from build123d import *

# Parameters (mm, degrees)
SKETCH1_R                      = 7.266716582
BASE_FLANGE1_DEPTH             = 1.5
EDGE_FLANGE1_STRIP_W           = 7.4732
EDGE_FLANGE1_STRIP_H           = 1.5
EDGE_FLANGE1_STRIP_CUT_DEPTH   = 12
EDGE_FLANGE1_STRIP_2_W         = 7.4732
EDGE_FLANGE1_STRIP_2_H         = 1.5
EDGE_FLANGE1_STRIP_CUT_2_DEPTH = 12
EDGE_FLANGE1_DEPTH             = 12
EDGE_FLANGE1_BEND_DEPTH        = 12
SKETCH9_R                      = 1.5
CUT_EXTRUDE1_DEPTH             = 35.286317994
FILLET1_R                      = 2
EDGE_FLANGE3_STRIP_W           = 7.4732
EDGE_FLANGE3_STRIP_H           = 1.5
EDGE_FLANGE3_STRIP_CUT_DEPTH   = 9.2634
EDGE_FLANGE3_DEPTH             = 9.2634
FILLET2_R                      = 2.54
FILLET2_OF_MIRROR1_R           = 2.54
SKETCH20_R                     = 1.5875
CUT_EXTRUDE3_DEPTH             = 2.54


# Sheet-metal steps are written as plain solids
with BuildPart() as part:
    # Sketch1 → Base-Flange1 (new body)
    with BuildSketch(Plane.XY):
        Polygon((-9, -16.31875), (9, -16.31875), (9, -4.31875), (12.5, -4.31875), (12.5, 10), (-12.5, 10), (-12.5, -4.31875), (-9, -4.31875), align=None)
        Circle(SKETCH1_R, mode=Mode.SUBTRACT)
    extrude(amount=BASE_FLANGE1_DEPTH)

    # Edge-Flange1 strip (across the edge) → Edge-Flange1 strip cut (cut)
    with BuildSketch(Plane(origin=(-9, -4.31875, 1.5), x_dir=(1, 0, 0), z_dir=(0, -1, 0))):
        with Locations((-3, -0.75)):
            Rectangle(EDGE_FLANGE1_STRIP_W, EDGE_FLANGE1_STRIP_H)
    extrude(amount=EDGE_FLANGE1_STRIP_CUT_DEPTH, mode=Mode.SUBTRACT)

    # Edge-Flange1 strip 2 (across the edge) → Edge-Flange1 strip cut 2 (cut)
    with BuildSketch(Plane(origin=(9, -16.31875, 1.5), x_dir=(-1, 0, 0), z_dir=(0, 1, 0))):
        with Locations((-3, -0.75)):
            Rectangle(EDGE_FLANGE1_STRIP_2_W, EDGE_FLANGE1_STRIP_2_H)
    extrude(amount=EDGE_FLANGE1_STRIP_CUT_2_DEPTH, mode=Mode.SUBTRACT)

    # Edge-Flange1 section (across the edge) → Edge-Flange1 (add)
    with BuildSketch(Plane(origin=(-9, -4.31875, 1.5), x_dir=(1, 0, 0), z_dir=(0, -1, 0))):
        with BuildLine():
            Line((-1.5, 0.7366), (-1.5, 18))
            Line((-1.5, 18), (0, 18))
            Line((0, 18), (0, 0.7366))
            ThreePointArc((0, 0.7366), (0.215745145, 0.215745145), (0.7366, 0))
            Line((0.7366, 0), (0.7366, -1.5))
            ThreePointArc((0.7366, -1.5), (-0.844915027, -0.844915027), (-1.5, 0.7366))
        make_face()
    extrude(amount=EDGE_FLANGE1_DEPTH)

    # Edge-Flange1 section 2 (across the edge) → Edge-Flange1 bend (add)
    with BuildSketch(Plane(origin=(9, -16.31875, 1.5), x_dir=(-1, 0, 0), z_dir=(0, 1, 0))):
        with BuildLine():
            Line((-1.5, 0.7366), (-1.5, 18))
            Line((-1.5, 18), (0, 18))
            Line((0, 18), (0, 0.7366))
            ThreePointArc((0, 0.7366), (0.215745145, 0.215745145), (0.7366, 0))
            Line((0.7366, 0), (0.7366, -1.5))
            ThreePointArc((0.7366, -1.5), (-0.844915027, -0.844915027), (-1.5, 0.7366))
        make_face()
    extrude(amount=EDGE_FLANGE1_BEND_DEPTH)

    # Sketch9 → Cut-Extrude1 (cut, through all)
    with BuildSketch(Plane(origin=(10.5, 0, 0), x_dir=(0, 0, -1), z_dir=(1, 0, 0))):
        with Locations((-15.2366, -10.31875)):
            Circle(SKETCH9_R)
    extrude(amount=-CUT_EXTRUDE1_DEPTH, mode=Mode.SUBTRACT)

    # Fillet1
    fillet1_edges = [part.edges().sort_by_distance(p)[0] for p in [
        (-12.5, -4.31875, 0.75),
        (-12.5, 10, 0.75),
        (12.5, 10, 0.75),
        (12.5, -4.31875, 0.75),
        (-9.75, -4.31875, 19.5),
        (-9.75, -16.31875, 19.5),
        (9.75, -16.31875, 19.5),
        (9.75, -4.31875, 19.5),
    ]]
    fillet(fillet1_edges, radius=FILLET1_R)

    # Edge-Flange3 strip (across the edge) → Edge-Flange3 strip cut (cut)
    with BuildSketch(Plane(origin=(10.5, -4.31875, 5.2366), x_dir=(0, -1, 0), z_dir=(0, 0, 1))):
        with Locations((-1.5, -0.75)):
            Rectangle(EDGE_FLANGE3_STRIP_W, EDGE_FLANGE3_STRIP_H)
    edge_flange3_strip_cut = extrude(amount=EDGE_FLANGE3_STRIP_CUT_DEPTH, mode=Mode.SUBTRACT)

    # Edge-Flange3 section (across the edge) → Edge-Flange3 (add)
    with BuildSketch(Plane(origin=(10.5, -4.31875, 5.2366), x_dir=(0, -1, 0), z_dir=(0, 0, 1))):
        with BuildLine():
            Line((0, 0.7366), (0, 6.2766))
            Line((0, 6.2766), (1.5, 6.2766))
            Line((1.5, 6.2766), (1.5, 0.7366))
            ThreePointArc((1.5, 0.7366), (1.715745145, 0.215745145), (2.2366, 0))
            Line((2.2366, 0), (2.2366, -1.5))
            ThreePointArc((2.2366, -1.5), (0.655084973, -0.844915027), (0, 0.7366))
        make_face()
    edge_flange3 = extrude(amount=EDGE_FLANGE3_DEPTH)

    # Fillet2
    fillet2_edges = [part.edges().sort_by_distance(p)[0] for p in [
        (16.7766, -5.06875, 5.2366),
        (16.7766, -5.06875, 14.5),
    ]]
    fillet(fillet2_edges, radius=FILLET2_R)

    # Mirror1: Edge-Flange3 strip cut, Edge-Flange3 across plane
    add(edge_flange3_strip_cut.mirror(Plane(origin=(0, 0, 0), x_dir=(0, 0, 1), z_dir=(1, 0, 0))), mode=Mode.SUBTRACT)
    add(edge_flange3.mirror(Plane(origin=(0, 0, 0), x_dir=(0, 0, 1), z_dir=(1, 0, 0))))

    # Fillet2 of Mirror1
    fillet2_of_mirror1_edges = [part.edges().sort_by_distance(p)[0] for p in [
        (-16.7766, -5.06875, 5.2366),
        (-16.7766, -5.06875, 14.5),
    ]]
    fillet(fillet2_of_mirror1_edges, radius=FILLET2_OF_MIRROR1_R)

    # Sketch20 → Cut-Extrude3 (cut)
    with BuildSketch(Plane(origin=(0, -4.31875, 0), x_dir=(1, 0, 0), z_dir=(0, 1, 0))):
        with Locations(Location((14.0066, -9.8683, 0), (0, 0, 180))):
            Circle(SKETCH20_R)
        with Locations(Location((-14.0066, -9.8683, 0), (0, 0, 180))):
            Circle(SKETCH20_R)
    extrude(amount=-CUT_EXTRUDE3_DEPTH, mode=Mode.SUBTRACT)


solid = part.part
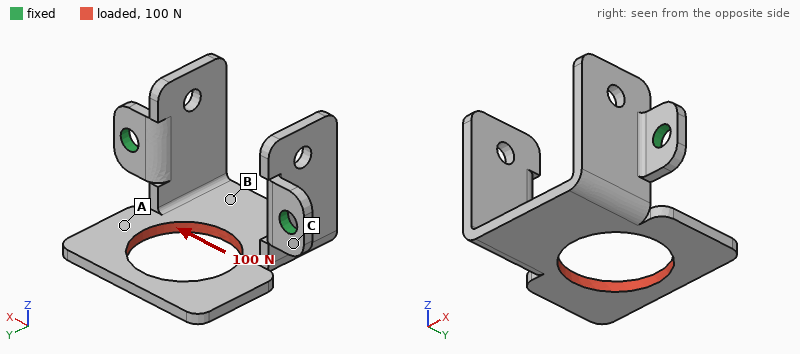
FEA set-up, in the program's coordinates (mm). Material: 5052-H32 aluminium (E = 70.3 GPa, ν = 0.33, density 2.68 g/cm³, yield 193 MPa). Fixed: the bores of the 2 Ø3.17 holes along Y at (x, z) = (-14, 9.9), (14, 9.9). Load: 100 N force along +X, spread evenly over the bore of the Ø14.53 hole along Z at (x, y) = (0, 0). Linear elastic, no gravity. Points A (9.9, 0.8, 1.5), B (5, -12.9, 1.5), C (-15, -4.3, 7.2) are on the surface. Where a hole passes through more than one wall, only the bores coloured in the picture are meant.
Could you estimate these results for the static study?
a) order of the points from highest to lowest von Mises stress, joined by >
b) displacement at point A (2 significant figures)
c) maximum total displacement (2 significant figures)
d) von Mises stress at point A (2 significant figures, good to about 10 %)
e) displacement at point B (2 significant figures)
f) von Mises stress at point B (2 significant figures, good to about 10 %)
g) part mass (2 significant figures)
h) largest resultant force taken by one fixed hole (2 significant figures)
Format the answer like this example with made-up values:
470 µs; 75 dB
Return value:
A > B > C; 44 µm; 66 µm; 25 MPa; 13 µm; 14 MPa; 3.7 g; 57 N
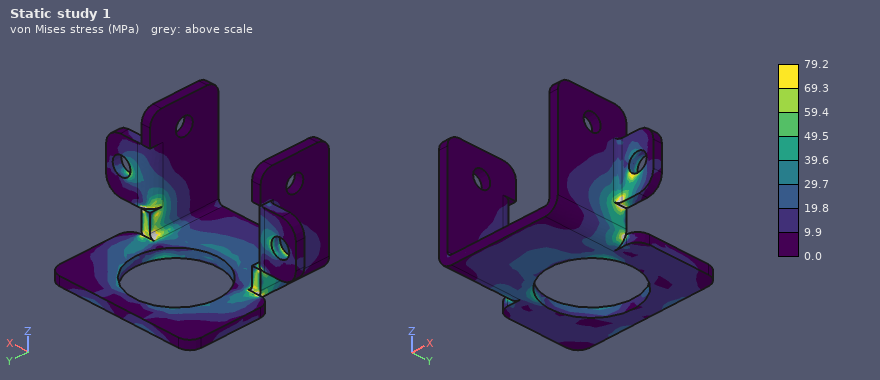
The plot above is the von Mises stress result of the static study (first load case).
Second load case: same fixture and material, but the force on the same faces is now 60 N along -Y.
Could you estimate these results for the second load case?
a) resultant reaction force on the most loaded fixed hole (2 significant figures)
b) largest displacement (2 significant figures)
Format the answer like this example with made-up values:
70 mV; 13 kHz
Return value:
31 N; 42 µm
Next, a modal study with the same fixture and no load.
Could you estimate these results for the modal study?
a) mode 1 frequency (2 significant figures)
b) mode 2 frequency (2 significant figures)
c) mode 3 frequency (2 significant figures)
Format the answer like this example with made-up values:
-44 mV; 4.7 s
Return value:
2800 Hz; 4900 Hz; 5200 Hz
